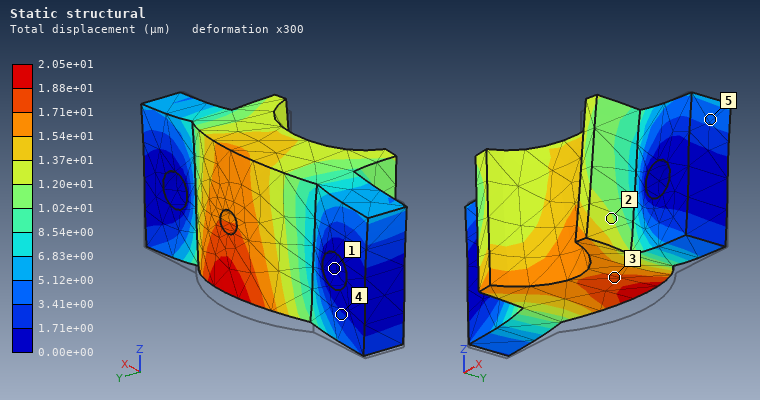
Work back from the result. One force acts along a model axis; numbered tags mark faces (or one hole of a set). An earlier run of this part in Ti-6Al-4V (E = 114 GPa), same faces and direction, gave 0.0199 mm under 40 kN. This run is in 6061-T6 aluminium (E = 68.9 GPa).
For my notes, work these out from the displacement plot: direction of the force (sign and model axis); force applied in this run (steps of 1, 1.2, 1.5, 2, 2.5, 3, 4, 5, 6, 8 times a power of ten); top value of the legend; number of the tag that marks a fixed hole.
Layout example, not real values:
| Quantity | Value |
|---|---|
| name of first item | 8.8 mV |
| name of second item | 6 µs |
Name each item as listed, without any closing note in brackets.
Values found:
| Quantity | Value |
|---|---|
| direction of the force | +Z |
| force applied in this run | 25 kN |
| top value of the legend | 2.05e+01 µm |
| number of the tag that marks a fixed hole | 1 |
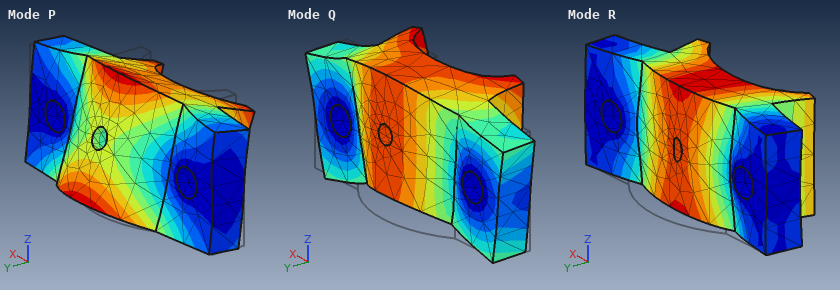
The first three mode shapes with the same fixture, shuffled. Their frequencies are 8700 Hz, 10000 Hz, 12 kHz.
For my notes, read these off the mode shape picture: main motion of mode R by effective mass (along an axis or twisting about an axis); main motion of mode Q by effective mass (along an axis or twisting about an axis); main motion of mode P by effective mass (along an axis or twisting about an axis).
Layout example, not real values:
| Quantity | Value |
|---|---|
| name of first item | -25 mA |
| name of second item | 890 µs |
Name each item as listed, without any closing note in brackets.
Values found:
| Quantity | Value |
|---|---|
| main motion of mode R by effective mass | along Y |
| main motion of mode Q by effective mass | along Z |
| main motion of mode P by effective mass | twisting about X |
